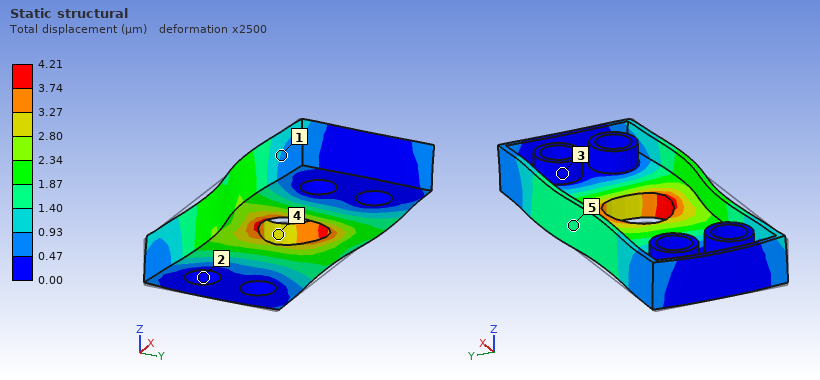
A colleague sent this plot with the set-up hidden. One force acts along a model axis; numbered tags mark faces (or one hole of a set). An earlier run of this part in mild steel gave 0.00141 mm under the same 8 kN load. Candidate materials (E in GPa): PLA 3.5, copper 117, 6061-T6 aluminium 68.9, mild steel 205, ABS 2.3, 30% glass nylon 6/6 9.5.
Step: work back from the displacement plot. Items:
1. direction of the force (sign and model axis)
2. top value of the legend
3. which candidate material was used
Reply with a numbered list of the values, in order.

1. +X
2. 4.21 µm
3. 6061-T6 aluminium
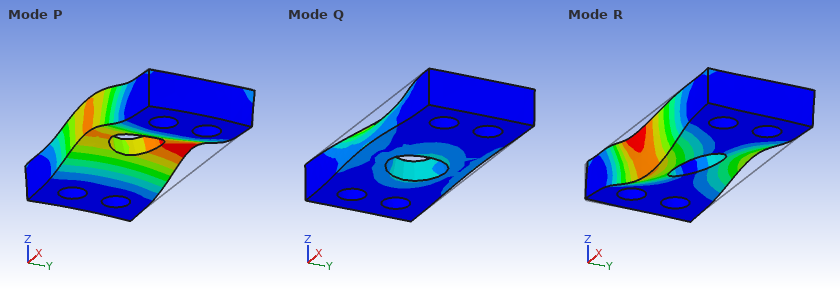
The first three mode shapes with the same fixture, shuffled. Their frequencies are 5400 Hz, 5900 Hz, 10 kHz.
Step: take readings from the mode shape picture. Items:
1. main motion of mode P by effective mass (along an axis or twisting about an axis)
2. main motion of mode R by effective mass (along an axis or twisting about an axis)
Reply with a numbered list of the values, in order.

1. along Z
2. twisting about X
